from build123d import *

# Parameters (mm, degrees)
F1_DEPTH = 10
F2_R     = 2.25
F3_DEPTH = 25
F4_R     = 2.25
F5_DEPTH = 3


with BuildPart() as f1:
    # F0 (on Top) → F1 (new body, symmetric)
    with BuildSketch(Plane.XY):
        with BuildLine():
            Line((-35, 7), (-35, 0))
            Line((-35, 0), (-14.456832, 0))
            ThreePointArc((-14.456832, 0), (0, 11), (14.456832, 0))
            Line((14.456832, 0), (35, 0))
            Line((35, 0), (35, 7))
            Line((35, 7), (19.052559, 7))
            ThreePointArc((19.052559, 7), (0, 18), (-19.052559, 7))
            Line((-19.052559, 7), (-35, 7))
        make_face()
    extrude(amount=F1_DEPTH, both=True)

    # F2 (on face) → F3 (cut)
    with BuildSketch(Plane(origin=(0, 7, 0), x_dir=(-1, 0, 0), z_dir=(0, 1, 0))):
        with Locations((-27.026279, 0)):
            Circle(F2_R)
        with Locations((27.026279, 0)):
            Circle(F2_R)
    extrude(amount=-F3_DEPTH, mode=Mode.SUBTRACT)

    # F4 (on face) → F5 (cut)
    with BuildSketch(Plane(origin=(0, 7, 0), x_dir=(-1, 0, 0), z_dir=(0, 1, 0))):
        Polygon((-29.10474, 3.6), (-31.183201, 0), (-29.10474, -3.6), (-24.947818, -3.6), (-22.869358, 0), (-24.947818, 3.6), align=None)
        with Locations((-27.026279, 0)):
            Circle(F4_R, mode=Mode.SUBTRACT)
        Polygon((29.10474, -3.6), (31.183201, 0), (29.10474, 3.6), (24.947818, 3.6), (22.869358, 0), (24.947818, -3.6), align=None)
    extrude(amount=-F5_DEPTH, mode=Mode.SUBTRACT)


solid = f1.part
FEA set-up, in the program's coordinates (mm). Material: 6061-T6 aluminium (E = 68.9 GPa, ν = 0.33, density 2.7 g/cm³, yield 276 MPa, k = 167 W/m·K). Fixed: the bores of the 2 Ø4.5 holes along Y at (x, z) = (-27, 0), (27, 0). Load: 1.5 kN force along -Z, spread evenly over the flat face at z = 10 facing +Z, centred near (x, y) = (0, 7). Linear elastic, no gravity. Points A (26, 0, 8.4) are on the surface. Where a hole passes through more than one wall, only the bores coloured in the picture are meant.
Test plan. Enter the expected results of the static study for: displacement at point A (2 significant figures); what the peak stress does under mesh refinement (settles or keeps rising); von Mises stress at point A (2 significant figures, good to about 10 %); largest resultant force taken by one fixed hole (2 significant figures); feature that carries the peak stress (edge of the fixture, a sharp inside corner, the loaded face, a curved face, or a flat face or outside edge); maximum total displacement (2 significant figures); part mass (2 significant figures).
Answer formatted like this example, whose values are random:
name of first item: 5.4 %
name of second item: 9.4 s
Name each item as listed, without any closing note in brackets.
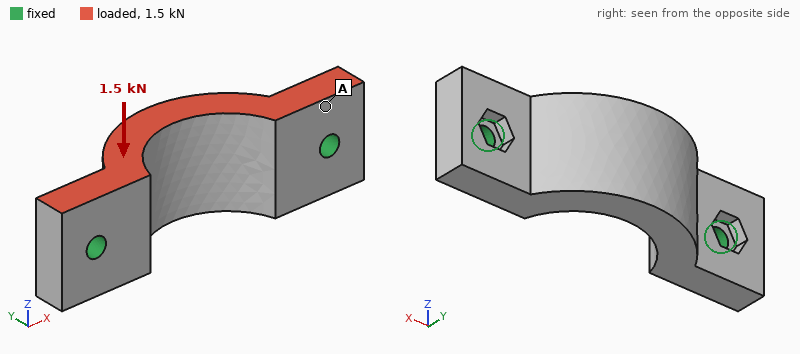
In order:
displacement at point A: 8.9 µm
what the peak stress does under mesh refinement: keeps rising
von Mises stress at point A: 13 MPa
largest resultant force taken by one fixed hole: 750 N
feature that carries the peak stress: edge of the fixture
maximum total displacement: 40 µm
part mass: 29 g
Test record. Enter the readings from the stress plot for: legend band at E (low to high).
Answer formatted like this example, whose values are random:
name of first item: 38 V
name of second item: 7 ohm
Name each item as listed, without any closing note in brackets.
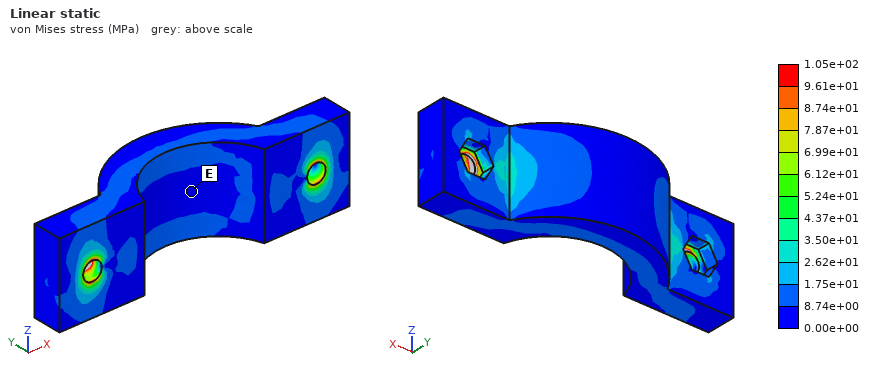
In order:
legend band at E: 0.00e+00 to 8.74e+00 MPa
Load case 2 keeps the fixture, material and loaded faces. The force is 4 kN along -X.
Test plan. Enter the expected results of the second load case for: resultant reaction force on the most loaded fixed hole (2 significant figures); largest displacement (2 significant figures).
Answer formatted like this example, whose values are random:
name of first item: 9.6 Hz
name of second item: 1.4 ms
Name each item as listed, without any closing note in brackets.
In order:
resultant reaction force on the most loaded fixed hole: 2.1 kN
largest displacement: 20 µm
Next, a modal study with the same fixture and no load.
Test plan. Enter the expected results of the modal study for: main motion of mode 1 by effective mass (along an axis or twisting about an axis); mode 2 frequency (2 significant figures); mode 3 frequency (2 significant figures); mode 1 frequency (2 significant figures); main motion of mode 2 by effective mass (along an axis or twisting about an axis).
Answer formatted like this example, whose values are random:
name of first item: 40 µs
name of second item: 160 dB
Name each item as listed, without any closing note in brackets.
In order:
main motion of mode 1 by effective mass: along Z
mode 2 frequency: 14 kHz
mode 3 frequency: 18 kHz
mode 1 frequency: 6700 Hz
main motion of mode 2 by effective mass: along Y
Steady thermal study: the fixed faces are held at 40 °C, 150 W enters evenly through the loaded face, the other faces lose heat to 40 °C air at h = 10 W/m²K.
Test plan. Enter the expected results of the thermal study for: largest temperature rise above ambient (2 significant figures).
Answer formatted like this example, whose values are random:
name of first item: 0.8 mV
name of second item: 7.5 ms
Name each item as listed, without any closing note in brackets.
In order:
largest temperature rise above ambient: 61 K
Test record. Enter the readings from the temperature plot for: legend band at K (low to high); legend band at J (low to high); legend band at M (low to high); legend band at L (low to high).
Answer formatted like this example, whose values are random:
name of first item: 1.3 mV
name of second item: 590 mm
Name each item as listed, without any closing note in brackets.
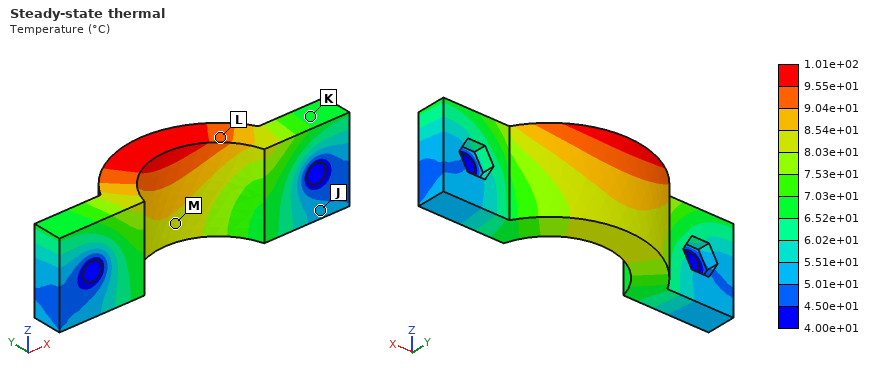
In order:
legend band at K: 6.52e+01 to 7.03e+01 °C
legend band at J: 5.01e+01 to 5.51e+01 °C
legend band at M: 8.03e+01 to 8.54e+01 °C
legend band at L: 9.04e+01 to 9.55e+01 °C
